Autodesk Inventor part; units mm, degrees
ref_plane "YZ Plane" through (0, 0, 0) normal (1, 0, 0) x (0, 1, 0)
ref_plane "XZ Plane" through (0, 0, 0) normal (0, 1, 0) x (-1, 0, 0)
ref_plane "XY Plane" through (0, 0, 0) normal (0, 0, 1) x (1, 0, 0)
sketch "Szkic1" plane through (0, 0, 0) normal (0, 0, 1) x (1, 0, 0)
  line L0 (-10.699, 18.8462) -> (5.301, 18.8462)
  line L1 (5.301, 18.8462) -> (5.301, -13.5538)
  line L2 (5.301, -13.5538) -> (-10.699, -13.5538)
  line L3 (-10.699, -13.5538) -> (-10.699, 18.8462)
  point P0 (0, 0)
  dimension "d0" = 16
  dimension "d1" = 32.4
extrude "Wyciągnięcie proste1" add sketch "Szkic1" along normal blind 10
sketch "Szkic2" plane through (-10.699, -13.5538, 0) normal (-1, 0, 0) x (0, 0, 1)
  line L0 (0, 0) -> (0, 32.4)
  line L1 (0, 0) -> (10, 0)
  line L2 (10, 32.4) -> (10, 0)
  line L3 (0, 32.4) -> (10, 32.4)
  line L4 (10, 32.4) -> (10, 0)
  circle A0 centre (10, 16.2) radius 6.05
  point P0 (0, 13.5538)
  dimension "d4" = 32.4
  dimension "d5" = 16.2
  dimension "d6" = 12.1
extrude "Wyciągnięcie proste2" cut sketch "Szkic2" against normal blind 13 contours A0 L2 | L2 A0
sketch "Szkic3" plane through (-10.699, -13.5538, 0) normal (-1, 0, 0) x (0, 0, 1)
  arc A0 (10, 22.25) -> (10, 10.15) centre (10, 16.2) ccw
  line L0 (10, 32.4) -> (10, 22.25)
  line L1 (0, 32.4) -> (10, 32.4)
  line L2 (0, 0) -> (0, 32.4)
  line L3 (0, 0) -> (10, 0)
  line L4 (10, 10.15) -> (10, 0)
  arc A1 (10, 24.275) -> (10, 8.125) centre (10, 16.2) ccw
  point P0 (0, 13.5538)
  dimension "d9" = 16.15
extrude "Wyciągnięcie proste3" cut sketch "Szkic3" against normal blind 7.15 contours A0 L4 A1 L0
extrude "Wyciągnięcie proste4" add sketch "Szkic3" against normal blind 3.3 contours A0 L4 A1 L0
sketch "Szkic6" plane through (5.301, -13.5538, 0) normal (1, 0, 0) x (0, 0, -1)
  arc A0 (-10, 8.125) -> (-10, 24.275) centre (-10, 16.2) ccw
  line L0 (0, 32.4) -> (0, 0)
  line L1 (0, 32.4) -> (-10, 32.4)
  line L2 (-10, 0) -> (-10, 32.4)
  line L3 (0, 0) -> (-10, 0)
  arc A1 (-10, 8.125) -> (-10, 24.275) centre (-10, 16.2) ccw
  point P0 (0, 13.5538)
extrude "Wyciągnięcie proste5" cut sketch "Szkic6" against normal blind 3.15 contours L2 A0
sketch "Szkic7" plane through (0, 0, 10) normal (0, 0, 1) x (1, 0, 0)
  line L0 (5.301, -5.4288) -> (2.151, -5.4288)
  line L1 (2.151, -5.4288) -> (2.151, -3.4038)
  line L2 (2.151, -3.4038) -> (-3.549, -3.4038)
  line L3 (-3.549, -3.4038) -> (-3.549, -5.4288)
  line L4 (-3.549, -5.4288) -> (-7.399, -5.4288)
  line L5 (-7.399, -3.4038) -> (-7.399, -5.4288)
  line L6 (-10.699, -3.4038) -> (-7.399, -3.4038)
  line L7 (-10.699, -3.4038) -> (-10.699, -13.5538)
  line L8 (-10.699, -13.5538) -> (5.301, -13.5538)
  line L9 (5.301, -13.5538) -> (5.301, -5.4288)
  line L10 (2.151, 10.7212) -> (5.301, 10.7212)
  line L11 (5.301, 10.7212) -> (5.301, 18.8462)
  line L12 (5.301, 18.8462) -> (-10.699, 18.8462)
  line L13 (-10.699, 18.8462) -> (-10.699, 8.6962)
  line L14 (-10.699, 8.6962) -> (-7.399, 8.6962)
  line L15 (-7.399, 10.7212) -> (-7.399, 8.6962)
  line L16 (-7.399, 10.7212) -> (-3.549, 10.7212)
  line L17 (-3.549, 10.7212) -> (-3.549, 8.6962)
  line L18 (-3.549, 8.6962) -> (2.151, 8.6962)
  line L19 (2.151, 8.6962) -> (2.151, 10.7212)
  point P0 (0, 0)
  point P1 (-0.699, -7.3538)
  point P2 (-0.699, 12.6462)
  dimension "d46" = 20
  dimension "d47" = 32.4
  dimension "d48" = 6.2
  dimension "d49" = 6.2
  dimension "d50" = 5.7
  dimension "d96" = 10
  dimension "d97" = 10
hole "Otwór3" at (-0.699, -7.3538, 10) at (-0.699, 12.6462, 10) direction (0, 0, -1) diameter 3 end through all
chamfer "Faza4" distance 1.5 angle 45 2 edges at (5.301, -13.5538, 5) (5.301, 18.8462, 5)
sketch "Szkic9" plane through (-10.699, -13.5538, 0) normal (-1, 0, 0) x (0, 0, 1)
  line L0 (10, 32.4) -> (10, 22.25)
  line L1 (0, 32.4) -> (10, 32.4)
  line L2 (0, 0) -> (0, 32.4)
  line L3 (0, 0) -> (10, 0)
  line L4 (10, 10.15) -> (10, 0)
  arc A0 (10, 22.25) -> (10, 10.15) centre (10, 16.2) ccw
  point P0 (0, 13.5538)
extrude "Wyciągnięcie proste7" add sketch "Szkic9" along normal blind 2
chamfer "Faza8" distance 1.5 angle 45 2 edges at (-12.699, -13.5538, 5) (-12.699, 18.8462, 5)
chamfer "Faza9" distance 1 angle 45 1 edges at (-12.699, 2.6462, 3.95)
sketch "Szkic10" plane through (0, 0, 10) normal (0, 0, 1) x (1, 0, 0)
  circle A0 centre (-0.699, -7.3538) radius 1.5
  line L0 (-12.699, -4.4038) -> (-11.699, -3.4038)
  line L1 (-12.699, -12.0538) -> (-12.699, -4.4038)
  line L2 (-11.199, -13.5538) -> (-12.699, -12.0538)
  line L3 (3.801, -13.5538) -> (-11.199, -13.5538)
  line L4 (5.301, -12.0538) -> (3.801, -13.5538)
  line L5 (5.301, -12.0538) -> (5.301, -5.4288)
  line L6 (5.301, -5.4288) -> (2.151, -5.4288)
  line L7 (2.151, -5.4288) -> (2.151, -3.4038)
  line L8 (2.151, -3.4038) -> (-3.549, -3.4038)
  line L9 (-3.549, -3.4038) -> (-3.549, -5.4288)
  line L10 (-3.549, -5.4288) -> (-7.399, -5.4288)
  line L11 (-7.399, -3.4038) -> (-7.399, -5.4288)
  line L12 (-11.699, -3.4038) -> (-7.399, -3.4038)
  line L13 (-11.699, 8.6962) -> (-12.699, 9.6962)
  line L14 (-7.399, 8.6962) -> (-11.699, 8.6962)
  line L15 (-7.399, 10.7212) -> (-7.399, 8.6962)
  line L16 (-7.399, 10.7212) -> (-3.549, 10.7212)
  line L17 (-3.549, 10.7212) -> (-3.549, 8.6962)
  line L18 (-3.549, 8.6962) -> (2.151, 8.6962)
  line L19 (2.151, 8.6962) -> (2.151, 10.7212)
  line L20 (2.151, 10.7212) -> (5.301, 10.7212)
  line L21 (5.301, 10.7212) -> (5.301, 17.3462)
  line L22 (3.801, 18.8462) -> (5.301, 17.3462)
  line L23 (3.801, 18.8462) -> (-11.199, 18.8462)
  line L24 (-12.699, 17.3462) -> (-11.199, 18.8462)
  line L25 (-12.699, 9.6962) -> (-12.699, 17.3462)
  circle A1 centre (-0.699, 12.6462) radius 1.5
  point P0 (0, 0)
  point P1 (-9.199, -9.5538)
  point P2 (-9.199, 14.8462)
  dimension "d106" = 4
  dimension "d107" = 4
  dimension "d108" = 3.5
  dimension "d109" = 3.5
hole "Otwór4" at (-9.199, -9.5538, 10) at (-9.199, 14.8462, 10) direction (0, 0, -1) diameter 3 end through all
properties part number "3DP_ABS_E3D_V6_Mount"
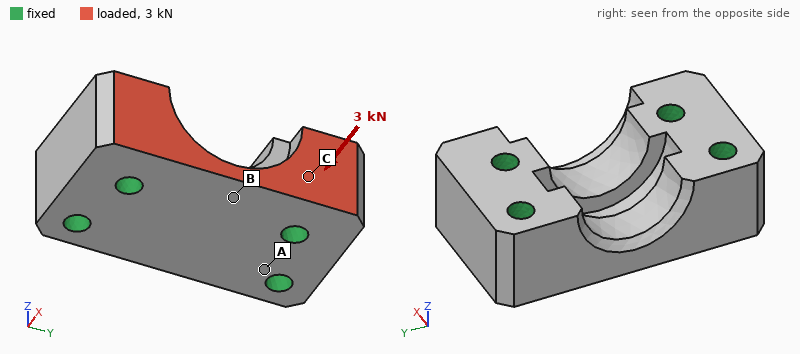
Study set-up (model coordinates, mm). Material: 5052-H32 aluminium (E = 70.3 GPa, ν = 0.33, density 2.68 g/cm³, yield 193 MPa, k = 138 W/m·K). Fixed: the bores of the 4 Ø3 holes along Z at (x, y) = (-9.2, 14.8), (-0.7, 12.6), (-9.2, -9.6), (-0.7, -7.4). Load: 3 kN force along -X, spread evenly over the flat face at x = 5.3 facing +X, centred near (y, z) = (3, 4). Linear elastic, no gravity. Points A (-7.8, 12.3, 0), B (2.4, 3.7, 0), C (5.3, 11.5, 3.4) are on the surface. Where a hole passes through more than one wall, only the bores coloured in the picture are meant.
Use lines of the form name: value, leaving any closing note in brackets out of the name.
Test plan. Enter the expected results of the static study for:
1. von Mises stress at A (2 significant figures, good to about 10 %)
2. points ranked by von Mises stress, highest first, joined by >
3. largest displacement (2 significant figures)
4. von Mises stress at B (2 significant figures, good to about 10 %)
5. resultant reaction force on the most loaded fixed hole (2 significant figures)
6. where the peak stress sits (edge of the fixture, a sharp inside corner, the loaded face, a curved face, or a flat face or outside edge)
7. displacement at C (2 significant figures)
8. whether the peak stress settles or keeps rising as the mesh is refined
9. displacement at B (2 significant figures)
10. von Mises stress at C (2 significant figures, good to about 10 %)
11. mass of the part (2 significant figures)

von Mises stress at A: 5.2 MPa
points ranked by von Mises stress, highest first, joined by >: C > B > A
largest displacement: 3.4 µm
von Mises stress at B: 12 MPa
resultant reaction force on the most loaded fixed hole: 1.3 kN
where the peak stress sits: edge of the fixture
displacement at C: 1.4 µm
whether the peak stress settles or keeps rising as the mesh is refined: keeps rising
displacement at B: 2.5 µm
von Mises stress at C: 19 MPa
mass of the part: 11 g
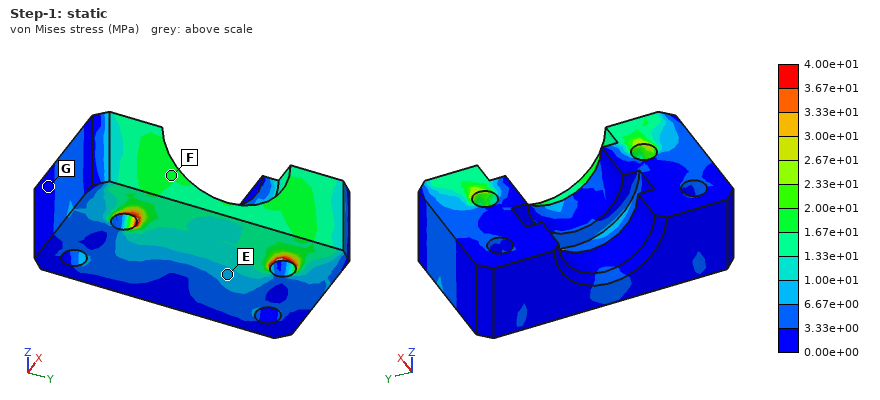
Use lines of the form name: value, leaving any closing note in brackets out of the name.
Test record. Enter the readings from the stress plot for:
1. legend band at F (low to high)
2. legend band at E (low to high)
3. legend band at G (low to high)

legend band at F: 1.67e+01 to 2.00e+01 MPa
legend band at E: 6.67e+00 to 1.00e+01 MPa
legend band at G: 0.00e+00 to 3.33e+00 MPa
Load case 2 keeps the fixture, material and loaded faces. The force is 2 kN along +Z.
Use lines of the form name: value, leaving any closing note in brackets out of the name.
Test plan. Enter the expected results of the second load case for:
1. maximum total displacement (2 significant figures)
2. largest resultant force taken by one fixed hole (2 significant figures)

maximum total displacement: 10 µm
largest resultant force taken by one fixed hole: 1.1 kN
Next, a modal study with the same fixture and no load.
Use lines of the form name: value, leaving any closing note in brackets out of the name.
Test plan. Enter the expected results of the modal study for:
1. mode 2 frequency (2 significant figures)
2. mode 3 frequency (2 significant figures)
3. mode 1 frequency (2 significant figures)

mode 2 frequency: 72 kHz
mode 3 frequency: 82 kHz
mode 1 frequency: 69 kHz
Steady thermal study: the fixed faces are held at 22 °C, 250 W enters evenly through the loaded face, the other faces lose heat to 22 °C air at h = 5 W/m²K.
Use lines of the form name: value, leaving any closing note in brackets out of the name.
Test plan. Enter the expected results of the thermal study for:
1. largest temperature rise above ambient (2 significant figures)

largest temperature rise above ambient: 63 K
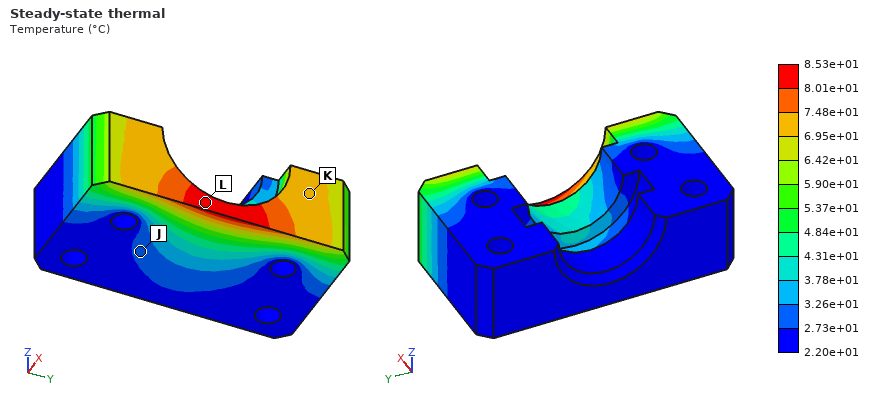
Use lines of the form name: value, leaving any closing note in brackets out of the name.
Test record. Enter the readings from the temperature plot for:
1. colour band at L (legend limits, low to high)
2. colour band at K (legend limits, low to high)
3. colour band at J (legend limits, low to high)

colour band at L: 8.01e+01 to 8.53e+01 °C
colour band at K: 6.95e+01 to 7.48e+01 °C
colour band at J: 2.73e+01 to 3.26e+01 °C
